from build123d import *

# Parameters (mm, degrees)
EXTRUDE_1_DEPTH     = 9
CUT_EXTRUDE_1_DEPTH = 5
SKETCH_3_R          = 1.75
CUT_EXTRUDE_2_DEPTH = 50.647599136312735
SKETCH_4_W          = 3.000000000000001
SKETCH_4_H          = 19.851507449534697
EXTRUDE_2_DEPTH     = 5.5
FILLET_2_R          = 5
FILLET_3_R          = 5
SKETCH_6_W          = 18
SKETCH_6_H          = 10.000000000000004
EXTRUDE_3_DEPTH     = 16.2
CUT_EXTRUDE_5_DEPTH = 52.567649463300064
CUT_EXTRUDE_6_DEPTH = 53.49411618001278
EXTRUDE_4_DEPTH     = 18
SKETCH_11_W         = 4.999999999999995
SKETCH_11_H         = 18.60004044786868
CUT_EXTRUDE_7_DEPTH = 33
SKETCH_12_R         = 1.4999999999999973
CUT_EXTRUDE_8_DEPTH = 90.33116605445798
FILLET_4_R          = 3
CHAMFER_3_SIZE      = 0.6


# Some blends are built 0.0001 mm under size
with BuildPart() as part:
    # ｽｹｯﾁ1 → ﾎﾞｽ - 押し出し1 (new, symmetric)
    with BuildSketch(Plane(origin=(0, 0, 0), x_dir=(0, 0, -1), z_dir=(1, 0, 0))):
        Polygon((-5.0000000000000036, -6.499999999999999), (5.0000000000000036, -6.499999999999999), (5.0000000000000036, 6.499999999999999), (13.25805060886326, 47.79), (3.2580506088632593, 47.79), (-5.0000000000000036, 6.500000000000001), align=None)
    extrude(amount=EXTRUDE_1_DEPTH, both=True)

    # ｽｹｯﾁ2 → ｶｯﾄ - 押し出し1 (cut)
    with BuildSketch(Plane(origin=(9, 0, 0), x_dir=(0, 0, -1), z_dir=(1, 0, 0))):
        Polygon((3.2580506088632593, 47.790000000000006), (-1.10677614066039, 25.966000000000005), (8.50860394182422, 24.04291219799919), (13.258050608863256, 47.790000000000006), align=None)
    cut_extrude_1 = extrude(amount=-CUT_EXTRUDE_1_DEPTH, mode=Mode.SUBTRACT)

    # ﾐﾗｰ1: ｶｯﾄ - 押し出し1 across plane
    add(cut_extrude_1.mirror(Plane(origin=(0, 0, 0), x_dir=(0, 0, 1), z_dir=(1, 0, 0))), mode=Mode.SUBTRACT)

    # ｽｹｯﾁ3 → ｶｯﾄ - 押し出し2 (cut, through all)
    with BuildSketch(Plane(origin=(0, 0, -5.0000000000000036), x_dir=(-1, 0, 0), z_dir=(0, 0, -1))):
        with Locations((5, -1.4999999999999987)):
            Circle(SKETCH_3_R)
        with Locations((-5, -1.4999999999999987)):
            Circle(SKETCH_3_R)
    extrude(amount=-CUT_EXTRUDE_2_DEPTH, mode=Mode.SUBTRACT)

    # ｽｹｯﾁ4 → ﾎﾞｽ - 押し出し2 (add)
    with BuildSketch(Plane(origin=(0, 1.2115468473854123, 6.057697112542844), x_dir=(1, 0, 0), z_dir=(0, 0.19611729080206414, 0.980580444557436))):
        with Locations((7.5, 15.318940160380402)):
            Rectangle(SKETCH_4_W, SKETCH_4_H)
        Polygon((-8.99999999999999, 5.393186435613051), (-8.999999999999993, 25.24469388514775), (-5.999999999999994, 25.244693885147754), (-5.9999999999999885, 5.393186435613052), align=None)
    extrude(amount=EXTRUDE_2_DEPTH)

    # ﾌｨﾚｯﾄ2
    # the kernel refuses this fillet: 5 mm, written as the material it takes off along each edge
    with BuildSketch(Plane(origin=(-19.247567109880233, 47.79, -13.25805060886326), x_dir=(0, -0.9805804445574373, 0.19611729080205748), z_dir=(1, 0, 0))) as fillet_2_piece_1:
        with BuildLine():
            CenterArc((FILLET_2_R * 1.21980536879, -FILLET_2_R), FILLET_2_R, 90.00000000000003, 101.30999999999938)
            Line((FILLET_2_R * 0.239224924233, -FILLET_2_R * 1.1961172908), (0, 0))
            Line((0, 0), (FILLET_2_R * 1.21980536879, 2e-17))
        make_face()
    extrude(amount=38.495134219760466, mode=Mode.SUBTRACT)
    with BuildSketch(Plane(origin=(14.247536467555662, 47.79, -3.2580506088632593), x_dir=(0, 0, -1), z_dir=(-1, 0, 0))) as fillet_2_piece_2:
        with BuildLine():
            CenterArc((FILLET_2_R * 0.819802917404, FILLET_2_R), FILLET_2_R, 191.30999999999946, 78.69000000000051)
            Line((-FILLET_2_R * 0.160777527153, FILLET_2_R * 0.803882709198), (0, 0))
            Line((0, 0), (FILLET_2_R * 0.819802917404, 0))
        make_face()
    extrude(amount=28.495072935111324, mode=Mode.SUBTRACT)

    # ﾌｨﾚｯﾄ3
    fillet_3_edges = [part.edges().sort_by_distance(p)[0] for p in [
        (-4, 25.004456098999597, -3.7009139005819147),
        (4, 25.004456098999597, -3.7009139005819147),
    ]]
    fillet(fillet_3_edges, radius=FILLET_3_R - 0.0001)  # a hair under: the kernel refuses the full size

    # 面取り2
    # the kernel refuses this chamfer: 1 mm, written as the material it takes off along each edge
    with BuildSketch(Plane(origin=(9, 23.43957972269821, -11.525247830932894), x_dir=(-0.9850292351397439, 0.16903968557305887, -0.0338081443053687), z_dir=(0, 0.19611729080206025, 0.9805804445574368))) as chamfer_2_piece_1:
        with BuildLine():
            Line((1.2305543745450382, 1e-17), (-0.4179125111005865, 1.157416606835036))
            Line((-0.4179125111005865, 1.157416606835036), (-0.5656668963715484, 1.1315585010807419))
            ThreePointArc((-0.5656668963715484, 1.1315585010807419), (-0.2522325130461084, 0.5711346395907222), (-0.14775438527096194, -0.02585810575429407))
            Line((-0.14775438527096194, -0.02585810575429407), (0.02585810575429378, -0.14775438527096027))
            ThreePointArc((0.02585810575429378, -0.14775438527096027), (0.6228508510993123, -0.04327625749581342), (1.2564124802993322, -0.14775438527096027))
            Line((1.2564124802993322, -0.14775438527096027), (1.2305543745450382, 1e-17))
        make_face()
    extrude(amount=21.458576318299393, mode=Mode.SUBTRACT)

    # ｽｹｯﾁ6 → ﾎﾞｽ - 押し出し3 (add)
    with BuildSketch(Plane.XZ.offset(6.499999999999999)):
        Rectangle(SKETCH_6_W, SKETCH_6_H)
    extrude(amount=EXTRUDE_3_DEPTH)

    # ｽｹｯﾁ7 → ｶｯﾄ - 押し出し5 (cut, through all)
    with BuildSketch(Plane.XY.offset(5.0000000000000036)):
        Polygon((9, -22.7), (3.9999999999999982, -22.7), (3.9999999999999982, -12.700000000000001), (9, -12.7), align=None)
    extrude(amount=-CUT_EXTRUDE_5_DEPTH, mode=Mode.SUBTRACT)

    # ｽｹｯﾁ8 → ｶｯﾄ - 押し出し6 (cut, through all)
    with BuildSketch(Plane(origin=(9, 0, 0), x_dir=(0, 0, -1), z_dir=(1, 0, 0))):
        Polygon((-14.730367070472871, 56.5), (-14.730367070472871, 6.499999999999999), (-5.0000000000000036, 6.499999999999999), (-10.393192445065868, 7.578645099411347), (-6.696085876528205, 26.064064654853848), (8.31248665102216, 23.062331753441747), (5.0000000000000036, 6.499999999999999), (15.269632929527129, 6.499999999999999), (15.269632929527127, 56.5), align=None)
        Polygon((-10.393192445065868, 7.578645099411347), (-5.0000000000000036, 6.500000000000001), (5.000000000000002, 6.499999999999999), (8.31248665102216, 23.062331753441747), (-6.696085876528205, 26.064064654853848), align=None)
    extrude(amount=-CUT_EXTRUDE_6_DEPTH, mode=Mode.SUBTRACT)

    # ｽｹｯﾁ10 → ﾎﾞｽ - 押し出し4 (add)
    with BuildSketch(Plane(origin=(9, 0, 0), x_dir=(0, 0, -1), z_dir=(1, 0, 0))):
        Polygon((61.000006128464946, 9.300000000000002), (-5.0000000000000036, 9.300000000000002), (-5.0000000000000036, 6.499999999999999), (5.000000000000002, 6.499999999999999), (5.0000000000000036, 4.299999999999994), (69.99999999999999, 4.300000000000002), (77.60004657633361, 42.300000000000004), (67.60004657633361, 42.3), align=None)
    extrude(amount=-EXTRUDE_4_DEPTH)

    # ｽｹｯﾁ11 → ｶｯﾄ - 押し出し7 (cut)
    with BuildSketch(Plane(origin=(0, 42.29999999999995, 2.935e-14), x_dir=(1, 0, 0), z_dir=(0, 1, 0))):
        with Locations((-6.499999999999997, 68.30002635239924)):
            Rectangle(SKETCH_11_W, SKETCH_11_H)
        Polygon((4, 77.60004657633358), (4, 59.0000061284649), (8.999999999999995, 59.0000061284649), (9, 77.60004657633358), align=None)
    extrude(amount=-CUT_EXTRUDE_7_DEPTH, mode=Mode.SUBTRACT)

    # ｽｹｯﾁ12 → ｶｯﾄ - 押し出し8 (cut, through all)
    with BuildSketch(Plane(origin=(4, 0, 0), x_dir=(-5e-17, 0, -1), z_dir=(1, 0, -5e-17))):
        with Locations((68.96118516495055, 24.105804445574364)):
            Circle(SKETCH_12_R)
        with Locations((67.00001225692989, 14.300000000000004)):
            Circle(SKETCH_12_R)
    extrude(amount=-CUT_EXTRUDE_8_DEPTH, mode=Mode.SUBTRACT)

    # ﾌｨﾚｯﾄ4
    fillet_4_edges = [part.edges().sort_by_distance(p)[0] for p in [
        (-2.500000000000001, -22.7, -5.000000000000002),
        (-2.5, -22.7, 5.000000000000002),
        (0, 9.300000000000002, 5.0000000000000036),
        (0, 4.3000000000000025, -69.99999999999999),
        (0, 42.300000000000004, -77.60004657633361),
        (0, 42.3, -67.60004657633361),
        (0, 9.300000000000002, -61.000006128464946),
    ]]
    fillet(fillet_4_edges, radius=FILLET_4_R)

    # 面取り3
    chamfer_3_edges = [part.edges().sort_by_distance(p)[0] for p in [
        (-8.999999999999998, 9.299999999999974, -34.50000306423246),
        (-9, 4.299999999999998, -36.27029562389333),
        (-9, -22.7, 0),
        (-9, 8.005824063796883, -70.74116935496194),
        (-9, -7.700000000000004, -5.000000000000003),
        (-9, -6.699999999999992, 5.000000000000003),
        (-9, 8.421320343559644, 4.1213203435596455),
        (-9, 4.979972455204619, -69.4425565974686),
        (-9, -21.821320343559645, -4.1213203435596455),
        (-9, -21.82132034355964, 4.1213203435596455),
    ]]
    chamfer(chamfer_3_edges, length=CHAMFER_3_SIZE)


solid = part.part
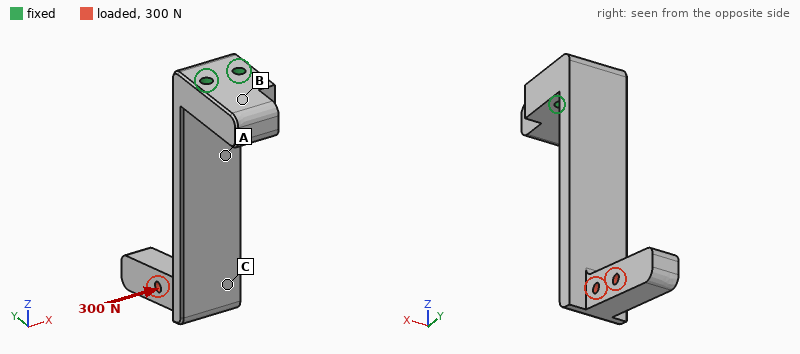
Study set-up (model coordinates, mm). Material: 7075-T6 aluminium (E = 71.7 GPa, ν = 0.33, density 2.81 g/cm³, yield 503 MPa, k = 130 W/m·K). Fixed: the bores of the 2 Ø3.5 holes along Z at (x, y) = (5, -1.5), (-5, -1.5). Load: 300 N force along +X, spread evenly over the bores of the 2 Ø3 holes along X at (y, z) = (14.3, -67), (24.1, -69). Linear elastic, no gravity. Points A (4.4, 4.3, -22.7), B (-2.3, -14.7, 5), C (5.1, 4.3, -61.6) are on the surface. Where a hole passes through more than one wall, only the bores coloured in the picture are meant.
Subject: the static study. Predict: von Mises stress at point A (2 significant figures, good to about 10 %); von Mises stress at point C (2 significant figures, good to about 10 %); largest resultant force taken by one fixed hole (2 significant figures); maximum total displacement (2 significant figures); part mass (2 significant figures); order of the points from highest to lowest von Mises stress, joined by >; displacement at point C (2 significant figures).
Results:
49 MPa
26 MPa
1.4 kN
0.71 mm
37 g
A > C > B
0.19 mm
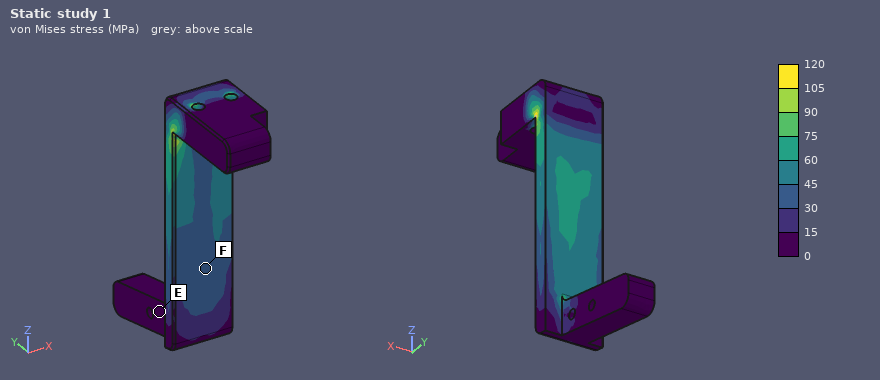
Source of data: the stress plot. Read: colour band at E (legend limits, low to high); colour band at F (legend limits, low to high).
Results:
0 to 15 MPa
30 to 45 MPa
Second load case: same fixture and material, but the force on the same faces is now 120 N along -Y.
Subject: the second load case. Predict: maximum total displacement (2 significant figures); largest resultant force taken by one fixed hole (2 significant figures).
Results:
1.2 mm
150 N
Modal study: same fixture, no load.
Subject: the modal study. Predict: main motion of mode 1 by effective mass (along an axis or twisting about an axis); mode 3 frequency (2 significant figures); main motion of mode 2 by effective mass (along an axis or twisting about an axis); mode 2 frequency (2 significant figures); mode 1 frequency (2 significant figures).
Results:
along Y
2400 Hz
along X
1200 Hz
510 Hz
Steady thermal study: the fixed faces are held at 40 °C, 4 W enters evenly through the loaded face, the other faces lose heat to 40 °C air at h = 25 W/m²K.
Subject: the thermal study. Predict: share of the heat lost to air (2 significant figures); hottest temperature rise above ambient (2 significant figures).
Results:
32 %
21 K
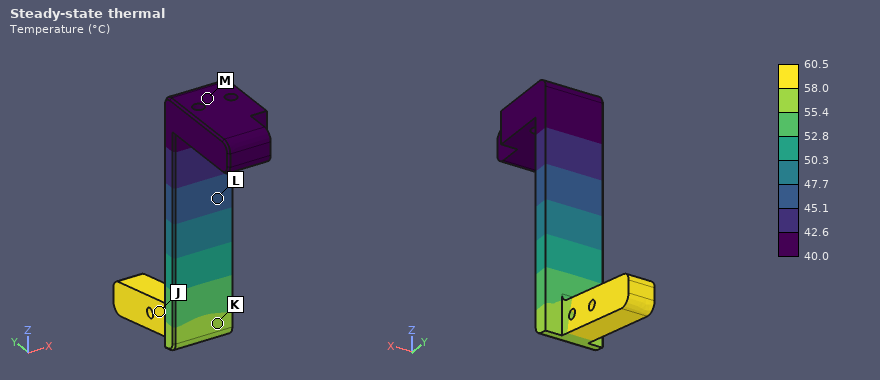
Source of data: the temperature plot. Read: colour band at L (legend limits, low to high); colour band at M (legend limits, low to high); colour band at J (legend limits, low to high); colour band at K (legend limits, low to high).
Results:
45.1 to 47.7 °C
40.0 to 42.6 °C
58.0 to 60.5 °C
55.4 to 58.0 °C
